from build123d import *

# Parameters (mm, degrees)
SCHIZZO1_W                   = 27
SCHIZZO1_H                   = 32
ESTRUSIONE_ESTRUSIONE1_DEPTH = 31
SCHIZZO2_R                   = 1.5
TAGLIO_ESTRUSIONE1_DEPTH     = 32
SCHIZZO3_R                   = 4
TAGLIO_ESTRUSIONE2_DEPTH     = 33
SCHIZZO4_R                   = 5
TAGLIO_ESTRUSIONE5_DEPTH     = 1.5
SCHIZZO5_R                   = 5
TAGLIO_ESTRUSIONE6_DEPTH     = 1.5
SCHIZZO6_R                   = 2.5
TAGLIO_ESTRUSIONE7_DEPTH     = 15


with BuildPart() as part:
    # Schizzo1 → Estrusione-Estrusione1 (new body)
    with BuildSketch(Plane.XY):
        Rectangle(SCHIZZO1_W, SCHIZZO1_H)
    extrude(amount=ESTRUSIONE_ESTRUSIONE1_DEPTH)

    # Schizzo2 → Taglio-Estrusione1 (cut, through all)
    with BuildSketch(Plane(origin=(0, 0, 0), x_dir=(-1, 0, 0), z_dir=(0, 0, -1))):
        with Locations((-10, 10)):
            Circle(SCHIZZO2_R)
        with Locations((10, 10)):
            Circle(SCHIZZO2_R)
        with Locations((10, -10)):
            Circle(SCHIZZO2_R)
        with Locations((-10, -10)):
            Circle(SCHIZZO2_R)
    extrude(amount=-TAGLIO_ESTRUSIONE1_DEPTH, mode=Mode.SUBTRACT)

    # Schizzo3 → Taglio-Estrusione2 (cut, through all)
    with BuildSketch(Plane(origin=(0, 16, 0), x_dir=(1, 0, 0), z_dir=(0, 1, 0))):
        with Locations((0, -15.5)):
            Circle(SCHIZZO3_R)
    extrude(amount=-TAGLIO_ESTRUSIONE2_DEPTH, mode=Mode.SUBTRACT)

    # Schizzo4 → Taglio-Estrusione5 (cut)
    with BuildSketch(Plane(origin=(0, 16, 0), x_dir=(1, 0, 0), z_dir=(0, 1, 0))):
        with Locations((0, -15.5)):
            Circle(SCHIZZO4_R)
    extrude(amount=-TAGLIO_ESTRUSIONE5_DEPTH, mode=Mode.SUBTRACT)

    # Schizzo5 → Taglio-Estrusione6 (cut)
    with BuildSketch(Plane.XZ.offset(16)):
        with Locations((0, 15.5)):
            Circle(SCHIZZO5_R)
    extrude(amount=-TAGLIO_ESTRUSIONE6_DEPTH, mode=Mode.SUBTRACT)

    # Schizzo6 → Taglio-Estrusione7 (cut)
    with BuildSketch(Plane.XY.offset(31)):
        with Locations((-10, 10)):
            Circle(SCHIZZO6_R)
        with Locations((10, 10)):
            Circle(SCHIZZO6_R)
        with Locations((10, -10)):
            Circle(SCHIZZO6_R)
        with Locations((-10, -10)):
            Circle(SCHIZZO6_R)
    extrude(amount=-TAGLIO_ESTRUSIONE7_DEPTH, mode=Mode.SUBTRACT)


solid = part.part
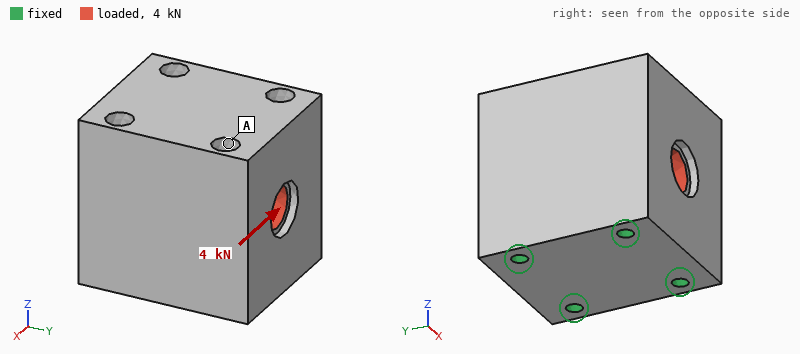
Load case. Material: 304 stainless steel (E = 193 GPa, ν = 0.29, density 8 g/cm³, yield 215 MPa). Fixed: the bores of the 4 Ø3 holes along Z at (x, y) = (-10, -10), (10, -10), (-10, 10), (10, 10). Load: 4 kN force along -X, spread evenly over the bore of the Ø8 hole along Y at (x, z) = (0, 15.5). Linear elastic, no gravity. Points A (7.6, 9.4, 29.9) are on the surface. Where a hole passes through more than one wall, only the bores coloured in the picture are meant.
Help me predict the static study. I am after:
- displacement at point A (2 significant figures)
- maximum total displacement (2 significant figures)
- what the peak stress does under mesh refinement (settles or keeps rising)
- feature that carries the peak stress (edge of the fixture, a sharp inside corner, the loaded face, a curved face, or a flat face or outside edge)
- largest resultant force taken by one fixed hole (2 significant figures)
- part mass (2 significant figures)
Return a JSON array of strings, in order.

["0.78 µm", "0.88 µm", "keeps rising", "edge of the fixture", "1.1 kN", "190 g"]
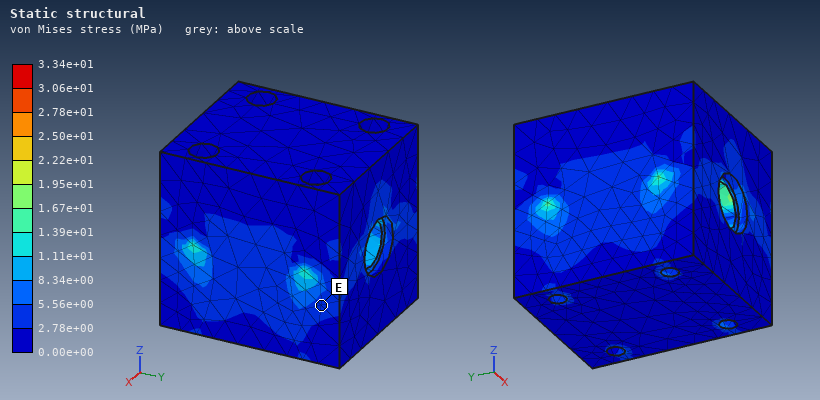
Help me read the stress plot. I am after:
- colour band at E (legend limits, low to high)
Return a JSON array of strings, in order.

["2.78e+00 to 5.56e+00 MPa"]
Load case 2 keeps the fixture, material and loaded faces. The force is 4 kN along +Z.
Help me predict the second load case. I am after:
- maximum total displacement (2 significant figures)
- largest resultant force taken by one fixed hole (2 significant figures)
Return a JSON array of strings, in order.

["0.62 µm", "1.0 kN"]
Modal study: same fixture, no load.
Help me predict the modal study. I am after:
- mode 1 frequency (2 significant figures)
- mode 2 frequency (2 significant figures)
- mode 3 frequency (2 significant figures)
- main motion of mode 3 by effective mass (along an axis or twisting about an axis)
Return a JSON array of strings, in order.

["24 kHz", "25 kHz", "33 kHz", "twisting about Z"]
